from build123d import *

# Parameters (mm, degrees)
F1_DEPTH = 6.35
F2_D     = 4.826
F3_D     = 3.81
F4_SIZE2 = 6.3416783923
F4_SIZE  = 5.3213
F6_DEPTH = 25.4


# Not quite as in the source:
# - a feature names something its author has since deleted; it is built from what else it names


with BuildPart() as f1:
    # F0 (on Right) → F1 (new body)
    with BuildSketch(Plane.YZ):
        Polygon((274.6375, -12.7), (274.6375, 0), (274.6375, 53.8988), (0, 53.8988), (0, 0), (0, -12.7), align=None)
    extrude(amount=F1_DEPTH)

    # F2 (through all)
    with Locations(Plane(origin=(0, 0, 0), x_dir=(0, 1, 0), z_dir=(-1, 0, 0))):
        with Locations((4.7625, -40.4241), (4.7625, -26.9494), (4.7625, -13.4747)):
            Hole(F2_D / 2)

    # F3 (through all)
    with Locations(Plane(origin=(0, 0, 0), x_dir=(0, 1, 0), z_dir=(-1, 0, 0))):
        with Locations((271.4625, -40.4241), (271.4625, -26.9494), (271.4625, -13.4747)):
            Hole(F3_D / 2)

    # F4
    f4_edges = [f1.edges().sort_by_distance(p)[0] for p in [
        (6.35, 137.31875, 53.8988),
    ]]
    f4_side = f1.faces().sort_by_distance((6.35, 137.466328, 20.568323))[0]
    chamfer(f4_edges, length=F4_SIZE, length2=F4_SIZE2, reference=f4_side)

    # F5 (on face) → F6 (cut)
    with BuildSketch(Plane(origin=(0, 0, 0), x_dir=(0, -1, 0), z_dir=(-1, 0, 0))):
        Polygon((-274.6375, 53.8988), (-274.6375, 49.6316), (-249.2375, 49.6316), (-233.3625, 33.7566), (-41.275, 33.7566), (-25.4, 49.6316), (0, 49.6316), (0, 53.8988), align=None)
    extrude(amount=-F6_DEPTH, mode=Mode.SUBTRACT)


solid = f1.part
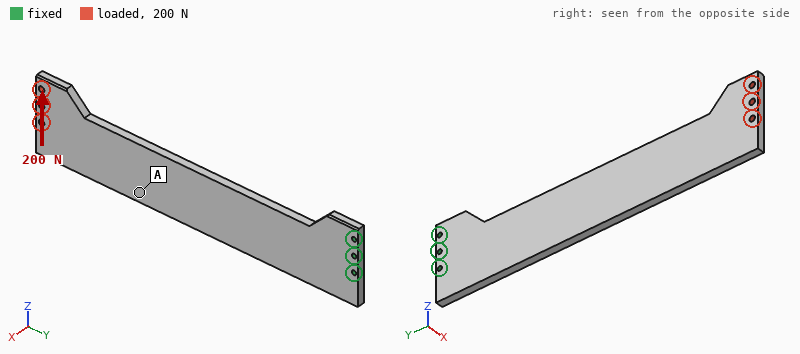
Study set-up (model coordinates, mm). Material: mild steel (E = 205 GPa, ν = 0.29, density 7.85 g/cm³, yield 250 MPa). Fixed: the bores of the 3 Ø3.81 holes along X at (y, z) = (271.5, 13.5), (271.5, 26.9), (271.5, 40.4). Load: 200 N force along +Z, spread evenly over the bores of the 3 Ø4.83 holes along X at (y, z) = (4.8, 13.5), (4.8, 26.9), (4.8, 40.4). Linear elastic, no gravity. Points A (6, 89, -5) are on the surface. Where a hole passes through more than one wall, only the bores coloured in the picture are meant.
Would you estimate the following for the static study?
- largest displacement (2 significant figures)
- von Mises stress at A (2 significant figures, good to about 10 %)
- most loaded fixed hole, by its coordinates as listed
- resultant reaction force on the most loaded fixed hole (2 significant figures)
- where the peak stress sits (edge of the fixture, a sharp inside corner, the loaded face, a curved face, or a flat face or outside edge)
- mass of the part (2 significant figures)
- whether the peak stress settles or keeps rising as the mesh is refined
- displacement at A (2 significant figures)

0.14 mm
5.0 MPa
(271.5, 13.5)
1.9 kN
edge of the fixture
680 g
keeps rising
0.076 mm
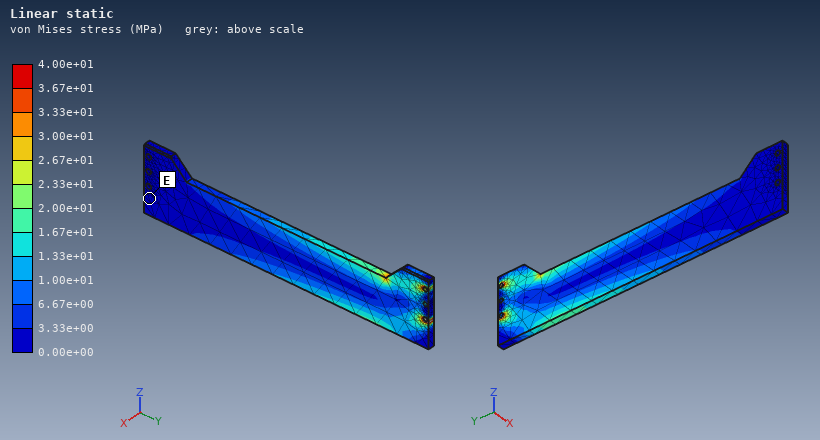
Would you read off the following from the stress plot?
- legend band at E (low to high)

0.00e+00 to 3.33e+00 MPa
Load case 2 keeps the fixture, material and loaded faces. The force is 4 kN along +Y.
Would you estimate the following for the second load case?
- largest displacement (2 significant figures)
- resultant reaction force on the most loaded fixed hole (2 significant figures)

0.20 mm
1.4 kN
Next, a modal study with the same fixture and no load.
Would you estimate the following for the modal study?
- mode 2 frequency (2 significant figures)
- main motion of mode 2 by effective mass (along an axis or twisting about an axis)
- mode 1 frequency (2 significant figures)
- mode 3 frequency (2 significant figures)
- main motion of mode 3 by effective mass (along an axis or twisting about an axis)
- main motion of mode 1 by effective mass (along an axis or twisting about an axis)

430 Hz
along X
68 Hz
450 Hz
along Z
along X
